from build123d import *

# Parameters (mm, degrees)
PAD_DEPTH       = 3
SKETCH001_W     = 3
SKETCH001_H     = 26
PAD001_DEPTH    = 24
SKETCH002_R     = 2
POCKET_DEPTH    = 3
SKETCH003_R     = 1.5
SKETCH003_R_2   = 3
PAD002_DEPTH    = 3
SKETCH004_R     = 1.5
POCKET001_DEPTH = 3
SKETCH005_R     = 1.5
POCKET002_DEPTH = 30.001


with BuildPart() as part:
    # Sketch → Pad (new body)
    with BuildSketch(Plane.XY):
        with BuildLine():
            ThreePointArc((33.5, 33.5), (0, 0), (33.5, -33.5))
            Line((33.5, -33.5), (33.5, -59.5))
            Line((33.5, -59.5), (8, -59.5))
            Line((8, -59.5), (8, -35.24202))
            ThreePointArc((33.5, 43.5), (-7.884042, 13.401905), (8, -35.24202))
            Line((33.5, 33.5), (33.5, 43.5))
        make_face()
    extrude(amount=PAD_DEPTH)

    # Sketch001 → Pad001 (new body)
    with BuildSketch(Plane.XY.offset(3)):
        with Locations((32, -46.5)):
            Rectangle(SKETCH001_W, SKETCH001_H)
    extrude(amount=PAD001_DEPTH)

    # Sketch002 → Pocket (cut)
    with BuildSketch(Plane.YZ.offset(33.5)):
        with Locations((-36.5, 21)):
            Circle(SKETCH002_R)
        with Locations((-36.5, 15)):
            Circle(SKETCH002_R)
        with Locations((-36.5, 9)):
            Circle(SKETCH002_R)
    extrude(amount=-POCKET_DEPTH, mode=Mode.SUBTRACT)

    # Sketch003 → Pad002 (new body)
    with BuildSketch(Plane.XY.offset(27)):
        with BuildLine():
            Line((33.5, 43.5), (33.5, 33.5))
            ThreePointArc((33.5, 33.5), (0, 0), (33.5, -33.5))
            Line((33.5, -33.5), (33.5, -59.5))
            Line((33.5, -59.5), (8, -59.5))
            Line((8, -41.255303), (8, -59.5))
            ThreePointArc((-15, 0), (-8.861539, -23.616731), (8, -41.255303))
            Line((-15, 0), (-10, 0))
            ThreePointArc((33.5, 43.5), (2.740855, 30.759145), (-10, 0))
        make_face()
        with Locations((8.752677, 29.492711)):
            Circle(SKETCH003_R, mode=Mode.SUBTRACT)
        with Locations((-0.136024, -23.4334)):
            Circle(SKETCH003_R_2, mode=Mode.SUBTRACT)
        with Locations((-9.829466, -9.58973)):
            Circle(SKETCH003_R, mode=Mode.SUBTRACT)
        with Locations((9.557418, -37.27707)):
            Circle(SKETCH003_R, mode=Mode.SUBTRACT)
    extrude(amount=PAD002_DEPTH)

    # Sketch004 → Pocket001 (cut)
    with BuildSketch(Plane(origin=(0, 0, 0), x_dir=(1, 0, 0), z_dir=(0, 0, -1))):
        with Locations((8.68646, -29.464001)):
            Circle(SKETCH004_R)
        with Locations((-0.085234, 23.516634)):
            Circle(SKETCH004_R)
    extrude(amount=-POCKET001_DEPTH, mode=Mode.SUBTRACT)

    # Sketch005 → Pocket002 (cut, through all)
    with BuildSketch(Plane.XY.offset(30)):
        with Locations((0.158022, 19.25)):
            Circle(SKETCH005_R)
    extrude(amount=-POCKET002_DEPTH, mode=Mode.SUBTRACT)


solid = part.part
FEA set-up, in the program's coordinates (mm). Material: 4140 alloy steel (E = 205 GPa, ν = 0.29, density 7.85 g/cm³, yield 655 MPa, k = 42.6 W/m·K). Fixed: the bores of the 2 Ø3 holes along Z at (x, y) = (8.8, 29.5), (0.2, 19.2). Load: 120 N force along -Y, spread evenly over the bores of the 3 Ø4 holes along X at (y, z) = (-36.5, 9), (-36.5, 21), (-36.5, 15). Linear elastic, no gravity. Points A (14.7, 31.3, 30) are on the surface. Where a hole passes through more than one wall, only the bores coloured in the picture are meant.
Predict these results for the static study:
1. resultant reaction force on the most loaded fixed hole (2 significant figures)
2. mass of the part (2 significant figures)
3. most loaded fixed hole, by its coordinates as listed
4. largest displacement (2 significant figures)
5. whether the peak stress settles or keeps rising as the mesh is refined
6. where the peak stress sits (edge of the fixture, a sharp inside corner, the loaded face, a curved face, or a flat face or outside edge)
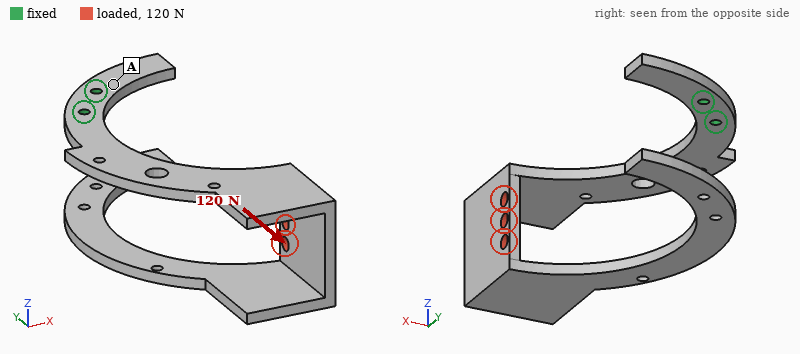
150 N
97 g
(8.8, 29.5)
1.3 mm
keeps rising
edge of the fixture
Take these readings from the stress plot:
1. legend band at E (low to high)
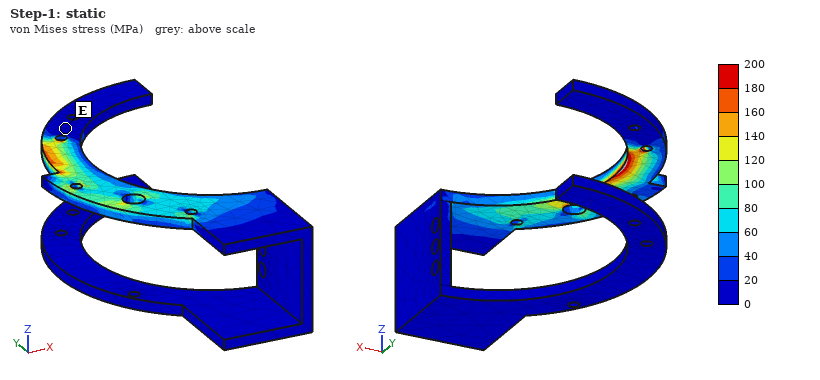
0 to 20 MPa
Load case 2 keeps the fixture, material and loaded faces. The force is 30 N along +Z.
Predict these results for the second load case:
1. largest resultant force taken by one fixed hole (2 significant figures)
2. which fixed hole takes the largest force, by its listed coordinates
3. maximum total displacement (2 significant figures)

40 N
(0.2, 19.2)
0.96 mm
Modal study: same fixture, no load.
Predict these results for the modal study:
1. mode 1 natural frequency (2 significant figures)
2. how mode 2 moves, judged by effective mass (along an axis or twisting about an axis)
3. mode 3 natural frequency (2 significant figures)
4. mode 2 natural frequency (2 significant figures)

120 Hz
along Z
230 Hz
190 Hz
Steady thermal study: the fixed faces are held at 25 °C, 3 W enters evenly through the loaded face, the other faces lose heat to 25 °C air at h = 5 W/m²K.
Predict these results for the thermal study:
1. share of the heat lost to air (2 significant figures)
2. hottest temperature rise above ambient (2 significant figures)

66 %
69 K
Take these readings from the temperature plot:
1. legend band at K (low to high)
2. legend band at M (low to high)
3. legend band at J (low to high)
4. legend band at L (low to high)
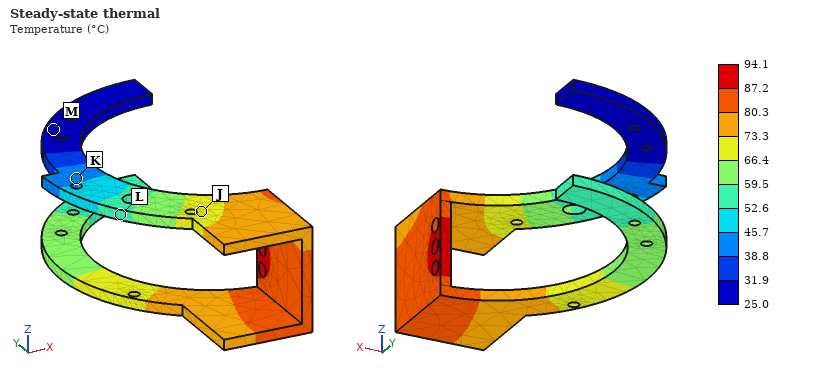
38.8 to 45.7 °C
25.0 to 31.9 °C
66.4 to 73.3 °C
52.6 to 59.5 °C
